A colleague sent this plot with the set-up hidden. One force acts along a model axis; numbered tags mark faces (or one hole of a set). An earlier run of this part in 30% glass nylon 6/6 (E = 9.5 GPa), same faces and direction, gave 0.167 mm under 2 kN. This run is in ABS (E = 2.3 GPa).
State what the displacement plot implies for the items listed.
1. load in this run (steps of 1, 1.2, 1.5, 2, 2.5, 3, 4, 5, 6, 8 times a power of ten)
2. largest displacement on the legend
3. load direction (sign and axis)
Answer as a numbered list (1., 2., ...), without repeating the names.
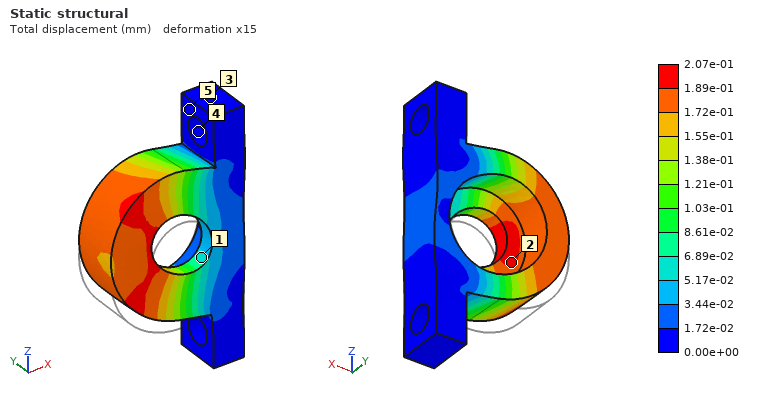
1. 600 N
2. 2.07e-01 mm
3. +Z
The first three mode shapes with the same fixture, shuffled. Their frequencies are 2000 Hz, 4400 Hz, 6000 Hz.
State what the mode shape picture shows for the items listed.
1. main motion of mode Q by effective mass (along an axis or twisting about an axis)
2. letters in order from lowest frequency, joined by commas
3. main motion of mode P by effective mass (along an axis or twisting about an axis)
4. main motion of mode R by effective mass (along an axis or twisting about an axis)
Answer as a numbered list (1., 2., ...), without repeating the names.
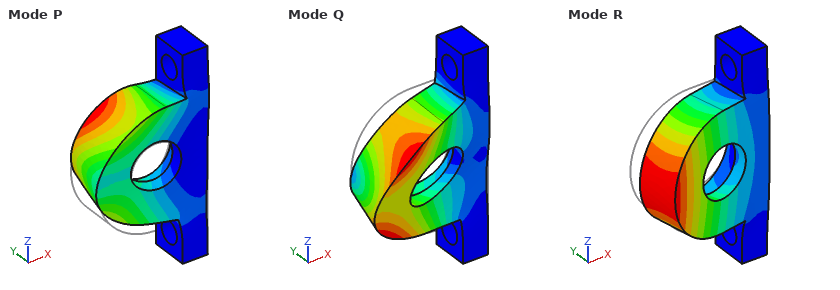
1. along Z
2. R, P, Q
3. along Z
4. along Y
